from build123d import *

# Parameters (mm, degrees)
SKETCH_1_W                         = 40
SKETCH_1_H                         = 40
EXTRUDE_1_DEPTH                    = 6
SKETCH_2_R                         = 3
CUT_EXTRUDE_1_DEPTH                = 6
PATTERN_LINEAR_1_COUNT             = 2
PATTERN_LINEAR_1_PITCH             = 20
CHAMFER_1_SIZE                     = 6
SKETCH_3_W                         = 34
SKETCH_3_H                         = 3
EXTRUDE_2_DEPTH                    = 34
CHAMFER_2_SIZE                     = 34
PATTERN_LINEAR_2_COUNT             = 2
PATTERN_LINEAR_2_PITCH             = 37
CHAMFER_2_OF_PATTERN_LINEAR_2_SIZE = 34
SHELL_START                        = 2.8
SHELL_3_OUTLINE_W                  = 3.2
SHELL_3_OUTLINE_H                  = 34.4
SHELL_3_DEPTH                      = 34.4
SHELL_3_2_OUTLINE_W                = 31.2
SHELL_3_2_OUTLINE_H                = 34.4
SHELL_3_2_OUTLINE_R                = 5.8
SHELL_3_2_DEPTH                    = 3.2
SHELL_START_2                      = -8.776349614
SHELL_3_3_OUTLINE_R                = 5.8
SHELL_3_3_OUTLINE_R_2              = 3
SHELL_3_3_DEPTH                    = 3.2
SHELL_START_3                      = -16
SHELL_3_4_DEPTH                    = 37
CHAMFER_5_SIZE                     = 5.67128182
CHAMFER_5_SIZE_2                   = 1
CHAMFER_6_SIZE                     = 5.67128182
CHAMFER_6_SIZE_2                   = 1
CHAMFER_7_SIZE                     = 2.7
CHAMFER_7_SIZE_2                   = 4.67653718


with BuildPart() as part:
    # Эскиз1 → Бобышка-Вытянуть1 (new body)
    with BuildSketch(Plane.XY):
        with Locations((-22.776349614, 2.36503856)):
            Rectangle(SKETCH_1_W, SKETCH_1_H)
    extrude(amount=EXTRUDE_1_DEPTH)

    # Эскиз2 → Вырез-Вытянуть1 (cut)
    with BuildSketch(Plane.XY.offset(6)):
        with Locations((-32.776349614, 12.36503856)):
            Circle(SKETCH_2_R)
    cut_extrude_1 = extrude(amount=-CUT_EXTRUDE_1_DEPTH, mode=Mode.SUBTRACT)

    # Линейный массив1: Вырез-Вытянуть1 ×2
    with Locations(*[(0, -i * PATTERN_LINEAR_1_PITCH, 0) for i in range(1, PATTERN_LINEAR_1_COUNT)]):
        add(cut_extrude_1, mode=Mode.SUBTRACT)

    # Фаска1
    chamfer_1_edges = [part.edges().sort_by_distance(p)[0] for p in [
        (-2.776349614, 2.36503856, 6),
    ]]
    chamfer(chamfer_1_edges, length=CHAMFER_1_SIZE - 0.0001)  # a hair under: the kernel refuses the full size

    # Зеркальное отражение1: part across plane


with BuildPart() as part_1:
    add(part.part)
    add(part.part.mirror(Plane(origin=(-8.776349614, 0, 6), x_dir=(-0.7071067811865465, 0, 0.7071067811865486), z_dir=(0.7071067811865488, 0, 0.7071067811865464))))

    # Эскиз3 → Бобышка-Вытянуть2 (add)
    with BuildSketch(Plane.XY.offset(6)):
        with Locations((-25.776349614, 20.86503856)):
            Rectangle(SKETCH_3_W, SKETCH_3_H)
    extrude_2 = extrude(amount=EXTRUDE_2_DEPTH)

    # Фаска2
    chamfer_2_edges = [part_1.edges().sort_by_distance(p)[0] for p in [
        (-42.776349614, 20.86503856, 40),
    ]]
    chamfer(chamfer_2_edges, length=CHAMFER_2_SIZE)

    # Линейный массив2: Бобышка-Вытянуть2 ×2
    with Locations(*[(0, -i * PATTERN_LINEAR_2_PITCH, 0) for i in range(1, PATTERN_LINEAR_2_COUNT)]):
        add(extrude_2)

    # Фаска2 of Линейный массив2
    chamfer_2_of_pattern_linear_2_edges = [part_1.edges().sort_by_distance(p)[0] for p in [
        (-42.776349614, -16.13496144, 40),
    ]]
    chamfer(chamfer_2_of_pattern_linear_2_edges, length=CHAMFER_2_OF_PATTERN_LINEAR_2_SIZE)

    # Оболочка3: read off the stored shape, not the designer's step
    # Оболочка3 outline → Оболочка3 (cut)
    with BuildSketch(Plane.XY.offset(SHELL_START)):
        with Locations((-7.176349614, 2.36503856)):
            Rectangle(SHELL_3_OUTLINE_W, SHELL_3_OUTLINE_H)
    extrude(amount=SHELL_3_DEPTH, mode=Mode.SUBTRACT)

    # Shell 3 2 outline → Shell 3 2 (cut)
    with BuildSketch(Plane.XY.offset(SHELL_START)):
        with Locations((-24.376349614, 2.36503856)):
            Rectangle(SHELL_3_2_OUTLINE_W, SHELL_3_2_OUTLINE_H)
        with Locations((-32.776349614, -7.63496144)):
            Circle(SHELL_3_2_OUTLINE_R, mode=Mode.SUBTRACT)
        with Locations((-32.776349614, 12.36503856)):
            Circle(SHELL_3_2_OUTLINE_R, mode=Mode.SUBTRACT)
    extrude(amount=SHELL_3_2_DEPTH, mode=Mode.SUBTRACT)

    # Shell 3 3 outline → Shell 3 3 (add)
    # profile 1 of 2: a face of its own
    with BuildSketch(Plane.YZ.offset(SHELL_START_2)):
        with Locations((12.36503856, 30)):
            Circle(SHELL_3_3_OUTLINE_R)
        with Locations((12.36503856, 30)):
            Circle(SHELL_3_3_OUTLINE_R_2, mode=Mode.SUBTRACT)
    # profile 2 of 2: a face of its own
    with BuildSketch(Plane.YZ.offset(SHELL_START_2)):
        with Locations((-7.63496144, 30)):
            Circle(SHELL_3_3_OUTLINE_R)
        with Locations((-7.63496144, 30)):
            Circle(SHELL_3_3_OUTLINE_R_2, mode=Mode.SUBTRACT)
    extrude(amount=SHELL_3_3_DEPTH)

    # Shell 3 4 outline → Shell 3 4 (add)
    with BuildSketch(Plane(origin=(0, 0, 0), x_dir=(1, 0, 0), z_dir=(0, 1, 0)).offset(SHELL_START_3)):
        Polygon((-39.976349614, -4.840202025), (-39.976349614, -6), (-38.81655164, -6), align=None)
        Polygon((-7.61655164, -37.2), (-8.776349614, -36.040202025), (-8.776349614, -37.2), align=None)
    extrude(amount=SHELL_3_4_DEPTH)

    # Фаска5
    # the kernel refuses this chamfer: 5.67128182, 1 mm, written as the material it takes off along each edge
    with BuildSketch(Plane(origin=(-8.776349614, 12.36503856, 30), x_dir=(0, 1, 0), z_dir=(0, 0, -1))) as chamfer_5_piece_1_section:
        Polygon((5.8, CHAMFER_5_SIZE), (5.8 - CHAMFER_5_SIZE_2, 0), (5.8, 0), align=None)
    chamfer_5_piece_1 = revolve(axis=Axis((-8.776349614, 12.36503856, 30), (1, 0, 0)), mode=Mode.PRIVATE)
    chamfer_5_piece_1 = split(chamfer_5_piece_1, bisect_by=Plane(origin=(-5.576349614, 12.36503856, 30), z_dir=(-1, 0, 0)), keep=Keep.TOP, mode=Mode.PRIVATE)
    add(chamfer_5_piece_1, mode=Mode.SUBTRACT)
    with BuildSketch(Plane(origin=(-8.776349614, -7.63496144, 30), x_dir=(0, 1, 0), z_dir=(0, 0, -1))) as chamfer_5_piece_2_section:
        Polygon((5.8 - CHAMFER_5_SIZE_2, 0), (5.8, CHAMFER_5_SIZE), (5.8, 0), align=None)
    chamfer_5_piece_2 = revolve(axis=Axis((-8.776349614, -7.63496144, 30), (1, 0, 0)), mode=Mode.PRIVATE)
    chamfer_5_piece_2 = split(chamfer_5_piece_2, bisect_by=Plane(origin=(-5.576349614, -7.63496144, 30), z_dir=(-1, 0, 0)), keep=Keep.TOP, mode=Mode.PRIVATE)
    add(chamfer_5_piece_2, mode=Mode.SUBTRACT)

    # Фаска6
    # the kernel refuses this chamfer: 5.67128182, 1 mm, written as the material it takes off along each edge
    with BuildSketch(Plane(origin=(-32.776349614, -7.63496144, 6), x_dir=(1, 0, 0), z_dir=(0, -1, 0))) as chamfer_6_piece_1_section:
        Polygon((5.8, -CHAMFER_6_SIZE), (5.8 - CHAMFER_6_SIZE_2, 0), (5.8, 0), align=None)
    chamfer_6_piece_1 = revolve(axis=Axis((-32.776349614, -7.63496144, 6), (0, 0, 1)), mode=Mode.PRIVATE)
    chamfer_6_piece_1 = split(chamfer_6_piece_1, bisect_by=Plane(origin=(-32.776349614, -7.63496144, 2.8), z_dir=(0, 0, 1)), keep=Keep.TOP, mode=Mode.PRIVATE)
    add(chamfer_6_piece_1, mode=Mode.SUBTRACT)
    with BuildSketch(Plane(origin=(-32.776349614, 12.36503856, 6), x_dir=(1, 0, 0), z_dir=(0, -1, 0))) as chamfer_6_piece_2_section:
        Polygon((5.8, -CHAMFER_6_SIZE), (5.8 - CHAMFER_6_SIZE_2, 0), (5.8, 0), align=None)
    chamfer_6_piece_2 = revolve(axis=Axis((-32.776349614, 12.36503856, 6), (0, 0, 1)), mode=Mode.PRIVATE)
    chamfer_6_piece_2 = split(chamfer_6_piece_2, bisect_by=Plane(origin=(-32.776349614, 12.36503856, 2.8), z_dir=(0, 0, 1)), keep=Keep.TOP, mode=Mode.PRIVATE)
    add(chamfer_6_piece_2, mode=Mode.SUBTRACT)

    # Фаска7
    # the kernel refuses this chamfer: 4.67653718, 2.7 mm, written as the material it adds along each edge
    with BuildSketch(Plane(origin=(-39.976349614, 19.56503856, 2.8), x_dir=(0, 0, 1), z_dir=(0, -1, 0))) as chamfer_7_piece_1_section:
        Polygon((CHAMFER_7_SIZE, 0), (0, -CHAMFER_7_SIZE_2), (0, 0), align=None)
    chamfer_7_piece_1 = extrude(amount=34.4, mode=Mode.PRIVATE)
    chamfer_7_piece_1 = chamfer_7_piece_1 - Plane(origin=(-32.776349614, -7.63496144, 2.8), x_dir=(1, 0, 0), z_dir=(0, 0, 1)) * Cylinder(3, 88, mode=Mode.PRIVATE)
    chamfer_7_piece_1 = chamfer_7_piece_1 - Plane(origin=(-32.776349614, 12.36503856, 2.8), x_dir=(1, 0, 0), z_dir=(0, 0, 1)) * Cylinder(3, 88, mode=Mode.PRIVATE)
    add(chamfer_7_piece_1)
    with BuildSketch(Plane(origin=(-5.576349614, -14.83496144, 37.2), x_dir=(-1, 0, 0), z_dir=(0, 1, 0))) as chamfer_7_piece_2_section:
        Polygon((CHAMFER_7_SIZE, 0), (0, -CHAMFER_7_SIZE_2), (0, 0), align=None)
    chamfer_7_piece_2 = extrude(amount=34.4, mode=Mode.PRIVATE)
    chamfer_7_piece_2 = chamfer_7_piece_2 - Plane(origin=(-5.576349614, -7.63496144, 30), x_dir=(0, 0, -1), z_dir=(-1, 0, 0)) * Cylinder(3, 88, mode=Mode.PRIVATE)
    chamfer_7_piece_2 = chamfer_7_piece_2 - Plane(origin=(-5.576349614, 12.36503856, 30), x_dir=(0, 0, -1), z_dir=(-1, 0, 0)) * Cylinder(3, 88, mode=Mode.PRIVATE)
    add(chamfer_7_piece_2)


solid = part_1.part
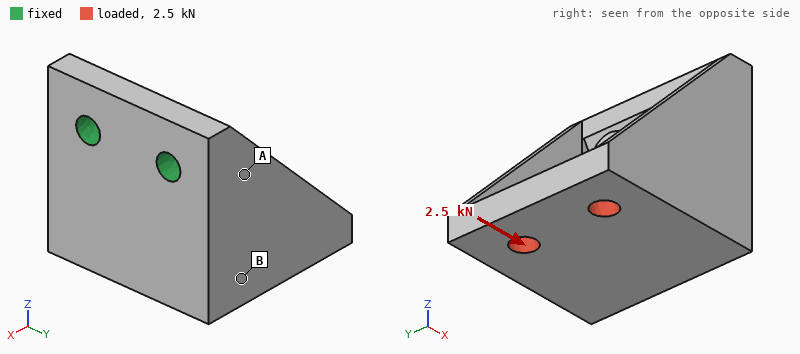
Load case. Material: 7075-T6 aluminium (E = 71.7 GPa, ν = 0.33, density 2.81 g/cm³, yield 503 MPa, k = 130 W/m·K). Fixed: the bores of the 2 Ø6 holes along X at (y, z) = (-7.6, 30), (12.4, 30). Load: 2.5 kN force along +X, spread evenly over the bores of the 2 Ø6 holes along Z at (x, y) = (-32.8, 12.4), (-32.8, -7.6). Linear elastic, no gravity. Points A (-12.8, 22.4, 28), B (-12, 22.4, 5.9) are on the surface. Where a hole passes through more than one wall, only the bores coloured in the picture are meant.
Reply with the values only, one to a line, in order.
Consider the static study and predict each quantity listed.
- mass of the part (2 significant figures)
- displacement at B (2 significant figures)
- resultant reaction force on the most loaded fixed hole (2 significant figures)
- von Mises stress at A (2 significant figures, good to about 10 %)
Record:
42 g
0.42 mm
1.3 kN
94 MPa
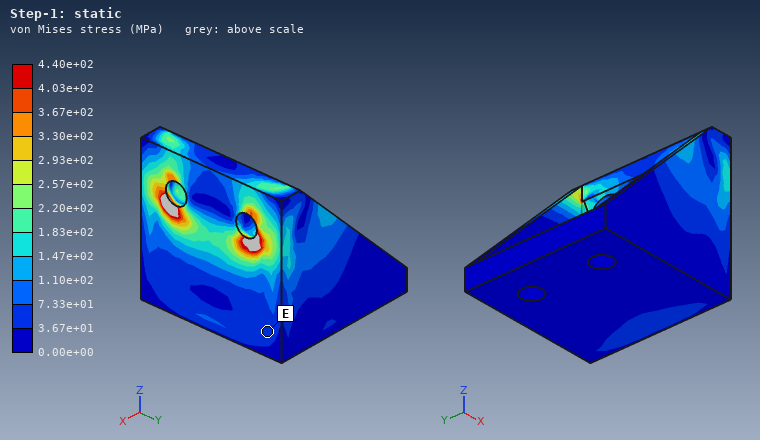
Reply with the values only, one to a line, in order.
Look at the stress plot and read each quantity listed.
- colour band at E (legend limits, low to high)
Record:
3.67e+01 to 7.33e+01 MPa
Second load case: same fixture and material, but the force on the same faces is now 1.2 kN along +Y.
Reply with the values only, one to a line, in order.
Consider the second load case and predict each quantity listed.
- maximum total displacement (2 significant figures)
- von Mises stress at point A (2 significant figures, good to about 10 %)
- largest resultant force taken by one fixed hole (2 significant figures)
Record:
0.70 mm
100 MPa
1.6 kN
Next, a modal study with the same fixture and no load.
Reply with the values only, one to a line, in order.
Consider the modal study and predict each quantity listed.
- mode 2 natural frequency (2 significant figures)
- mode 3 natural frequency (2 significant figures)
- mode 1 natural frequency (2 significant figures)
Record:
1900 Hz
6700 Hz
1800 Hz
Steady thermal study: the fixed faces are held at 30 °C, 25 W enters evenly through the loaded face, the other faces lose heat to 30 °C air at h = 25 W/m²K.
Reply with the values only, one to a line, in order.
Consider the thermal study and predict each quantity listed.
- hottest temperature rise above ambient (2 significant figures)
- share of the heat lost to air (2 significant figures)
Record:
44 K
20 %
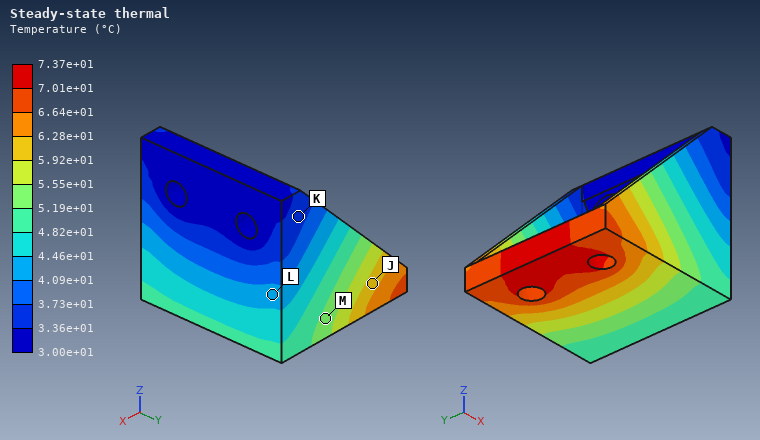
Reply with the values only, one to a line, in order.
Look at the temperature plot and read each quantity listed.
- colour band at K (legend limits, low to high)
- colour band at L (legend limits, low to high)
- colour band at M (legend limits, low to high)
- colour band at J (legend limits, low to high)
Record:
3.36e+01 to 3.73e+01 °C
4.09e+01 to 4.46e+01 °C
5.19e+01 to 5.55e+01 °C
5.92e+01 to 6.28e+01 °C
